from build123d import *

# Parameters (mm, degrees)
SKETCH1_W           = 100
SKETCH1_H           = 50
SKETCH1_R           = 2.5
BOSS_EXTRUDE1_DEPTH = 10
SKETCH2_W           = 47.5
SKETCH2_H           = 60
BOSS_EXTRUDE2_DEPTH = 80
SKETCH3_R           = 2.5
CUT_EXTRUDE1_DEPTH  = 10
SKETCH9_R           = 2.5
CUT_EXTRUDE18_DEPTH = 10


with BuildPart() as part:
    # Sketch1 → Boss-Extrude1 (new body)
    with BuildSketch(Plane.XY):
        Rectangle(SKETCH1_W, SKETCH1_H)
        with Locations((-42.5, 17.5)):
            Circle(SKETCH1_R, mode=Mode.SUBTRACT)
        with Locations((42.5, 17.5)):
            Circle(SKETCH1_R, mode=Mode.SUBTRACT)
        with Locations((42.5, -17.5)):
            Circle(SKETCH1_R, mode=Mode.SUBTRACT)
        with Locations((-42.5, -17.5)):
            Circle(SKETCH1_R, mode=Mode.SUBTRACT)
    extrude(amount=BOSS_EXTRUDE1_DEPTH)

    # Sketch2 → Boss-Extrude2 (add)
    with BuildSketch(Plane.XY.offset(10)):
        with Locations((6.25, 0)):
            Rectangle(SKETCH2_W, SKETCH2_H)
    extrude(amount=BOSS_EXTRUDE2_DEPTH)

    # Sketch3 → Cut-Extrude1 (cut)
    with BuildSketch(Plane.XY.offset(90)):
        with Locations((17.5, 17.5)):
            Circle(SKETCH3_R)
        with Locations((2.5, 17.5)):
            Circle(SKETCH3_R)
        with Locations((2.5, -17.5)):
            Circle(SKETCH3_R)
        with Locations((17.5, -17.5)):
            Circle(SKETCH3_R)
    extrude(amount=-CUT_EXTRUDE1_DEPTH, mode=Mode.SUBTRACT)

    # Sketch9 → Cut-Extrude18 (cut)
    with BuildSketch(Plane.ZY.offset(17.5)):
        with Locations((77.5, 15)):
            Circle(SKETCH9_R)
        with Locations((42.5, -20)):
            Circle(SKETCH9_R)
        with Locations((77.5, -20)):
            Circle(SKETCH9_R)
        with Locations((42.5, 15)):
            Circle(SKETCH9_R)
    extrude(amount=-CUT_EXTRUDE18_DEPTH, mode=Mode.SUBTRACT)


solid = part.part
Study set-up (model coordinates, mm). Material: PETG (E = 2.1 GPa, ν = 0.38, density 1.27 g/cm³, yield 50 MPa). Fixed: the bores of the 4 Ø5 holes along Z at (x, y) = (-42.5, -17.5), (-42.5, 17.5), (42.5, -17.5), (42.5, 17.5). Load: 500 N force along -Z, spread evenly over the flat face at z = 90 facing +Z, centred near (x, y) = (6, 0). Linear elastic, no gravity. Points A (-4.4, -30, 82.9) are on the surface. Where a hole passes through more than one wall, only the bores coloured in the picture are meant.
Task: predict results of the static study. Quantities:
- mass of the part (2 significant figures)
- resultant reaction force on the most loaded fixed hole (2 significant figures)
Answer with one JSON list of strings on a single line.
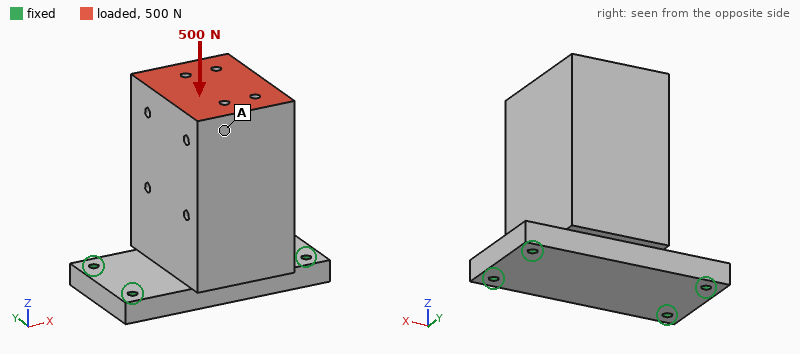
["350 g", "150 N"]
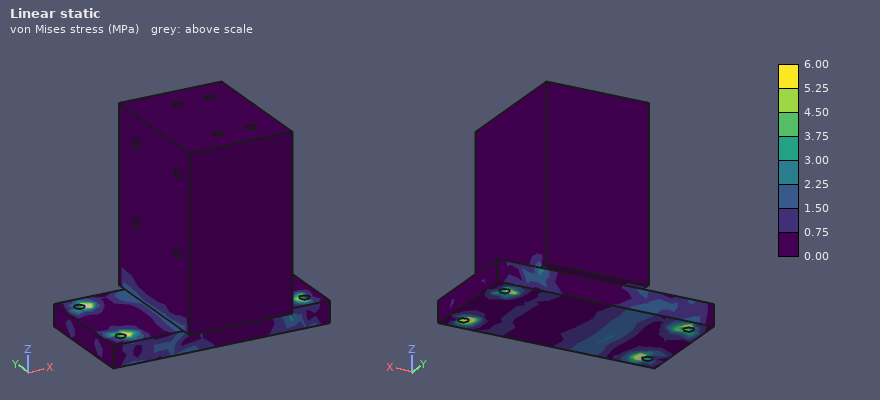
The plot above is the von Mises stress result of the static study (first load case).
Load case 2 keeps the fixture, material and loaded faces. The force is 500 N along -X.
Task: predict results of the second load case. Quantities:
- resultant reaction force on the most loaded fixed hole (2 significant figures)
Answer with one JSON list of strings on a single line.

["340 N"]
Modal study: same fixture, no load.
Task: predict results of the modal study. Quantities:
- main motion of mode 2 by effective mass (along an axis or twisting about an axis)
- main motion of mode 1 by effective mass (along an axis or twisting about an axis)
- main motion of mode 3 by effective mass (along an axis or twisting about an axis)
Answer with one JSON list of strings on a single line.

["along X", "along Y", "along Z"]
